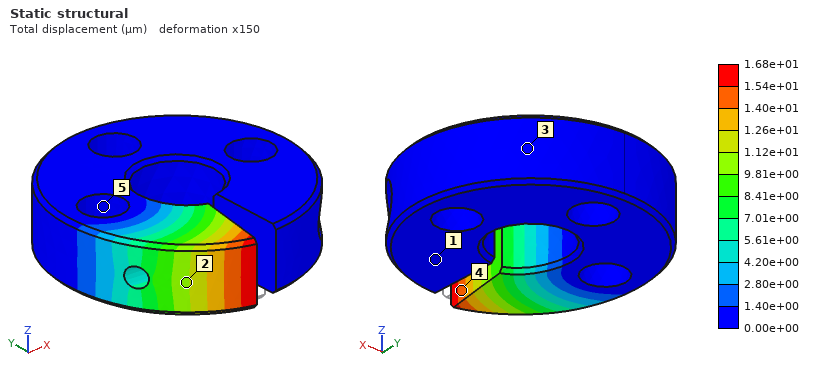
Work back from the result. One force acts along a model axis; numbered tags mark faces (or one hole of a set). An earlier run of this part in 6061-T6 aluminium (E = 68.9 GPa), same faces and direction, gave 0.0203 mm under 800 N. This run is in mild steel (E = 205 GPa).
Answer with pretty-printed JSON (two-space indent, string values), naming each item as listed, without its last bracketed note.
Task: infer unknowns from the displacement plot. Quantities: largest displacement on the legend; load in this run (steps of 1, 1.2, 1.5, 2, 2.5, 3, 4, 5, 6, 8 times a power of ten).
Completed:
{
  "largest displacement on the legend": "1.68e+01 µm",
  "load in this run": "2 kN"
}
